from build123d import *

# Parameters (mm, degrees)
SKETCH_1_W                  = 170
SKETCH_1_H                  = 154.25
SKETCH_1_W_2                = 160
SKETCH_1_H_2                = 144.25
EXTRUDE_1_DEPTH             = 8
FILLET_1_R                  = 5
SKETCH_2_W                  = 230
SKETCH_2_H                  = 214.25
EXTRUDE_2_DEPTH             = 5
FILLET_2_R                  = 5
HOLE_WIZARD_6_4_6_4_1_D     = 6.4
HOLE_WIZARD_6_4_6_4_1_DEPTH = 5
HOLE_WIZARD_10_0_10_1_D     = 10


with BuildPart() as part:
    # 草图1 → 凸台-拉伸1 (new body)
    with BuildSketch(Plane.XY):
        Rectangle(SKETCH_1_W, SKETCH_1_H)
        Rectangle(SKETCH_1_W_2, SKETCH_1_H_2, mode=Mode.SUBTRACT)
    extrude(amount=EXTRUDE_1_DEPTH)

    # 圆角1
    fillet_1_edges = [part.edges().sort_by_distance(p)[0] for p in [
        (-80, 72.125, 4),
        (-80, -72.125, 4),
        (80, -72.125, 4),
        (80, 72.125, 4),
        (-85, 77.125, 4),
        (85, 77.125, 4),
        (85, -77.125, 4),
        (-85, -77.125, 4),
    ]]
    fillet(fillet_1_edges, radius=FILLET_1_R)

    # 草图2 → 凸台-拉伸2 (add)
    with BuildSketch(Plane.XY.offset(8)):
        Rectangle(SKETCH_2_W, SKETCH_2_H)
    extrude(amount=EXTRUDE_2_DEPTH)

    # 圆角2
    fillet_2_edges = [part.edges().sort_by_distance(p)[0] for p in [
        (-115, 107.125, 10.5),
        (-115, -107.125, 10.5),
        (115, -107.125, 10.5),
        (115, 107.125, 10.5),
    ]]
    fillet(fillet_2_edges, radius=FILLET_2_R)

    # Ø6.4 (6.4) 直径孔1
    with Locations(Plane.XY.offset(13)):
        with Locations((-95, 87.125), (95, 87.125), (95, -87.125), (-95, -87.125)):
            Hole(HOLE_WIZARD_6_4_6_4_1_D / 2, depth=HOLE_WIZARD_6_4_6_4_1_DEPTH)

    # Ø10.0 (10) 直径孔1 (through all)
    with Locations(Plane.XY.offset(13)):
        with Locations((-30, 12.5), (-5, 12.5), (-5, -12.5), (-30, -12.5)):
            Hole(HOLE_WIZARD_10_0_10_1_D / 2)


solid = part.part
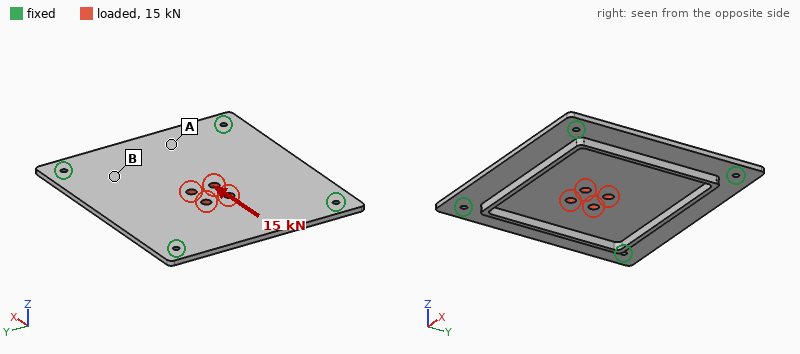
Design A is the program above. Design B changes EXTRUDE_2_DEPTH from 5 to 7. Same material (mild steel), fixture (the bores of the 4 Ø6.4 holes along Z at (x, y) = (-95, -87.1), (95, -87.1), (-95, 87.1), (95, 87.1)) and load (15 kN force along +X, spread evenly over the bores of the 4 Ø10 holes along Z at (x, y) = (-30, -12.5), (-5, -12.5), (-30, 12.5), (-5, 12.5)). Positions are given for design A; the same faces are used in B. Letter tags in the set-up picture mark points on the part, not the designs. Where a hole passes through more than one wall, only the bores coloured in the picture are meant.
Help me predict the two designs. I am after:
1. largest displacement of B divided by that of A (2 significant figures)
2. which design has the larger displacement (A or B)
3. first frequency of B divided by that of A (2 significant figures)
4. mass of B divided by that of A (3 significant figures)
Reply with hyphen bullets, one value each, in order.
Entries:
- 0.71
- A
- 1.2
- 1.36
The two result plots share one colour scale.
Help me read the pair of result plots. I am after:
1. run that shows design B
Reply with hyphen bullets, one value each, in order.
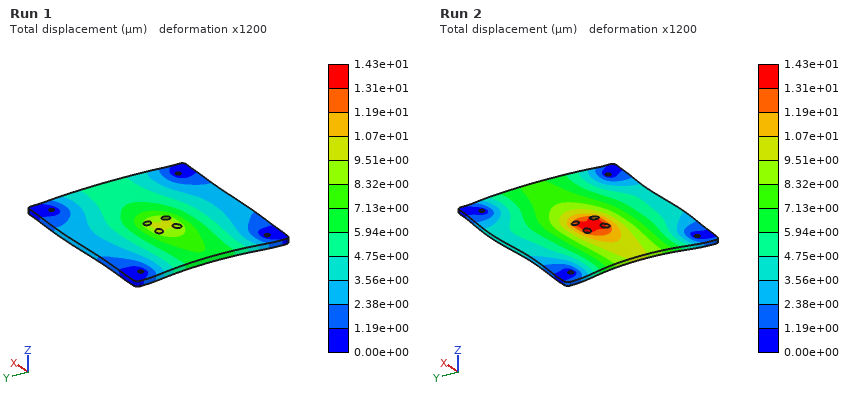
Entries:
- Run 1
